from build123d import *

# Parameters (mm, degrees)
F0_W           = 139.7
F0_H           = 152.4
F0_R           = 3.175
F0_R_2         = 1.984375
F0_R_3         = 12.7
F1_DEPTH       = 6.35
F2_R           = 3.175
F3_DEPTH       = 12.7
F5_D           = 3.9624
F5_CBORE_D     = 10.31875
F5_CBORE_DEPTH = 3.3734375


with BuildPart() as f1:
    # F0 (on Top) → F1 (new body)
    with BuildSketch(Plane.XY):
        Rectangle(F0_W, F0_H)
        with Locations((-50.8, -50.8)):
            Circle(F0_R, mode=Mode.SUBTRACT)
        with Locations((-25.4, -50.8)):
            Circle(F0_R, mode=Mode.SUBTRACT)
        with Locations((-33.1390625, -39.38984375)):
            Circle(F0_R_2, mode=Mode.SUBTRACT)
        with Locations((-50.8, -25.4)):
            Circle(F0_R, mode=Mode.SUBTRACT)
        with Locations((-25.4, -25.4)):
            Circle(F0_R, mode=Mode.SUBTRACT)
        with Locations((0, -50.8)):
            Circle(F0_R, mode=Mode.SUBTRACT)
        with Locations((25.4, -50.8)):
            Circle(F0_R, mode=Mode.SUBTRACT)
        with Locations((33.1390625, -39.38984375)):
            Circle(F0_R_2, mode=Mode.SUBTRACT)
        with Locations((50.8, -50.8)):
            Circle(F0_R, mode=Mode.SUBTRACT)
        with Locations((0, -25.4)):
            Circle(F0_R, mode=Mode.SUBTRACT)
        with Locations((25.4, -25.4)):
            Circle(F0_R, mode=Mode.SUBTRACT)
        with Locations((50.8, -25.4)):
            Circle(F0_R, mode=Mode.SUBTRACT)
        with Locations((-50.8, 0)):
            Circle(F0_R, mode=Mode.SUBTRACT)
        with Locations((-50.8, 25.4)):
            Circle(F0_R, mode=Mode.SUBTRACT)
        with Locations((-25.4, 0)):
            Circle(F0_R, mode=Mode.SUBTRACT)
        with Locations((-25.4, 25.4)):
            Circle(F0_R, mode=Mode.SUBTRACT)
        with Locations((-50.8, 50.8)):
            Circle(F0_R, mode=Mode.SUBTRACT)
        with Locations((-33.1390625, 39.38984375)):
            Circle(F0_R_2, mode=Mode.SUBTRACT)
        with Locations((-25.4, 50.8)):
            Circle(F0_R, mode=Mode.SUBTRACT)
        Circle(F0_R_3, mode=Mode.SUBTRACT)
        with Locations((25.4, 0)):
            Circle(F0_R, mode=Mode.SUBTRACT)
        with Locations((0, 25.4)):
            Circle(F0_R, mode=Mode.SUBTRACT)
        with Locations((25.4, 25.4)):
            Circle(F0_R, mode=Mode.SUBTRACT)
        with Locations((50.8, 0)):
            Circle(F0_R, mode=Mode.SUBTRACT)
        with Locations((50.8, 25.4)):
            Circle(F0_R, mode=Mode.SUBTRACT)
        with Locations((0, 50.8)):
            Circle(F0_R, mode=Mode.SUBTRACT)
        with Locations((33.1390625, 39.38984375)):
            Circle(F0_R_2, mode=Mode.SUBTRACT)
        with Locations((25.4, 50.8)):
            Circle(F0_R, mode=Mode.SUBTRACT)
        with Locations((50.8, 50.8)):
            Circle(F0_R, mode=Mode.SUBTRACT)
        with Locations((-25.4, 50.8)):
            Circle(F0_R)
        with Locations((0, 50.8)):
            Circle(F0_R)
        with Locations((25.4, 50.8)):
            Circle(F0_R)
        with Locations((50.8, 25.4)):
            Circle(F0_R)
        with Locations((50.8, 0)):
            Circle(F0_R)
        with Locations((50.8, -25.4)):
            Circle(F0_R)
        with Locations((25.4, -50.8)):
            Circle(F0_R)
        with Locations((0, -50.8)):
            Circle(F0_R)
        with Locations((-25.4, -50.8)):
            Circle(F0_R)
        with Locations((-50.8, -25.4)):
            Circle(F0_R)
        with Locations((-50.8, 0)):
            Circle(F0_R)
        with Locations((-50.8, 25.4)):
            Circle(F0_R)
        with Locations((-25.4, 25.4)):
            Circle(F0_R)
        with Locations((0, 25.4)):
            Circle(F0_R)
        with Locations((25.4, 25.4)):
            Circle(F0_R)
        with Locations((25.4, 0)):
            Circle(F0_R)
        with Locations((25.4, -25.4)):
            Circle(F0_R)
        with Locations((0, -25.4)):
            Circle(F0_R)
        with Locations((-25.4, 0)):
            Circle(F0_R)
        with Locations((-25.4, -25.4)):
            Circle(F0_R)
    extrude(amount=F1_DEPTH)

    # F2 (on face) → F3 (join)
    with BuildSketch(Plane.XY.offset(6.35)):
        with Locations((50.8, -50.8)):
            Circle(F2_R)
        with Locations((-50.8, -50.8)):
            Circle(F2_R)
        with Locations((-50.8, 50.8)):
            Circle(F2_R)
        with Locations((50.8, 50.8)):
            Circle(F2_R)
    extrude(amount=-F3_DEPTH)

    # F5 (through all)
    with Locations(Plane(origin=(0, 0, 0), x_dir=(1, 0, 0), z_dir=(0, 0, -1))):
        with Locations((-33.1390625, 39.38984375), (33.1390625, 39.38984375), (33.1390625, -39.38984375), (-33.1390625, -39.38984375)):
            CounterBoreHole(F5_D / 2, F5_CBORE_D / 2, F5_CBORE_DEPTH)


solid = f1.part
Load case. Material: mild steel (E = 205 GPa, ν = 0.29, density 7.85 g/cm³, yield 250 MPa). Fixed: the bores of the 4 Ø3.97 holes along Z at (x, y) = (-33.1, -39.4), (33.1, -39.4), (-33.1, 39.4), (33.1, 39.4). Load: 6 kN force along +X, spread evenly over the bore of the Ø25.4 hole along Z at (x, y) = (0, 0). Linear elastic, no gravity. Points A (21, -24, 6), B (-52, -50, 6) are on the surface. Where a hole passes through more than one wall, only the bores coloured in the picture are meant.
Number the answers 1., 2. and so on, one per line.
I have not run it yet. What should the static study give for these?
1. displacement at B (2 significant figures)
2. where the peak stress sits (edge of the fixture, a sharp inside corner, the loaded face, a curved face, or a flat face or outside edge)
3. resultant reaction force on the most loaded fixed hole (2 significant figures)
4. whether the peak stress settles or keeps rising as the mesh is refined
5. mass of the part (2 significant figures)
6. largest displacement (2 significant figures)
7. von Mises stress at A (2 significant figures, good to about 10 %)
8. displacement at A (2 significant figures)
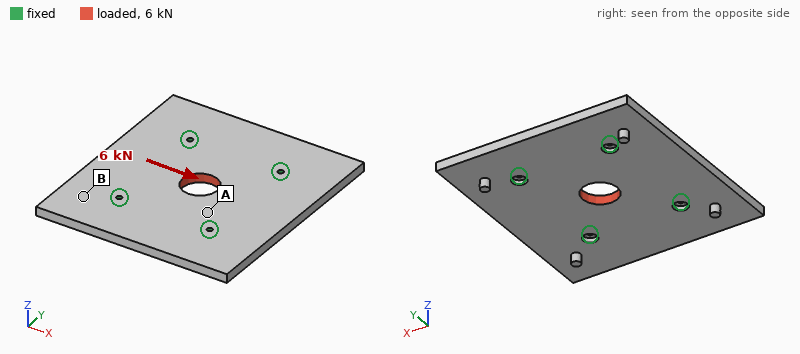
1. 2.1 µm
2. edge of the fixture
3. 1.5 kN
4. keeps rising
5. 1.0 kg
6. 3.8 µm
7. 9.5 MPa
8. 1.9 µm
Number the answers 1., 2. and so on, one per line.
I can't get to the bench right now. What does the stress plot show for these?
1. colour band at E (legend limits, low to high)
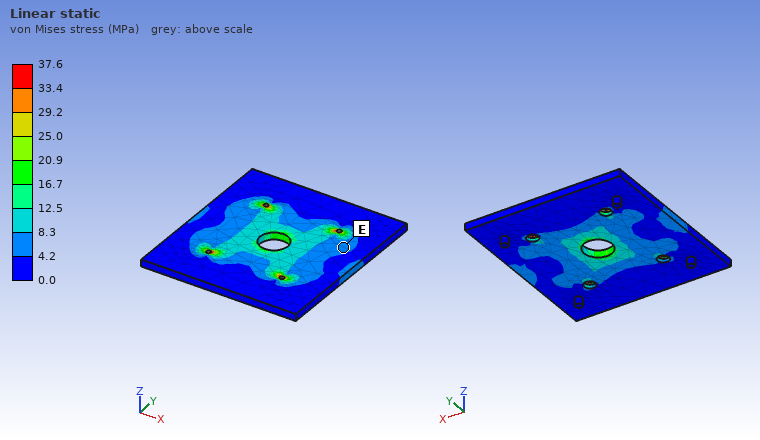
1. 4.2 to 8.3 MPa
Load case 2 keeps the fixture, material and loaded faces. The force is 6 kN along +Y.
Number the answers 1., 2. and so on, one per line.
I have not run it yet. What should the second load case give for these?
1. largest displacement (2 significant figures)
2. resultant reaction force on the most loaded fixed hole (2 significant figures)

1. 4.1 µm
2. 1.5 kN
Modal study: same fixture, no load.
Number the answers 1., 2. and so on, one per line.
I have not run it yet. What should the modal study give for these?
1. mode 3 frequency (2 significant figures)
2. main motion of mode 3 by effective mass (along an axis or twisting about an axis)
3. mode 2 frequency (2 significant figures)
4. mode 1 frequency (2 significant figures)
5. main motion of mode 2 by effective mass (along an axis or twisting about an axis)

1. 2300 Hz
2. twisting about Y
3. 2000 Hz
4. 1900 Hz
5. along Z
